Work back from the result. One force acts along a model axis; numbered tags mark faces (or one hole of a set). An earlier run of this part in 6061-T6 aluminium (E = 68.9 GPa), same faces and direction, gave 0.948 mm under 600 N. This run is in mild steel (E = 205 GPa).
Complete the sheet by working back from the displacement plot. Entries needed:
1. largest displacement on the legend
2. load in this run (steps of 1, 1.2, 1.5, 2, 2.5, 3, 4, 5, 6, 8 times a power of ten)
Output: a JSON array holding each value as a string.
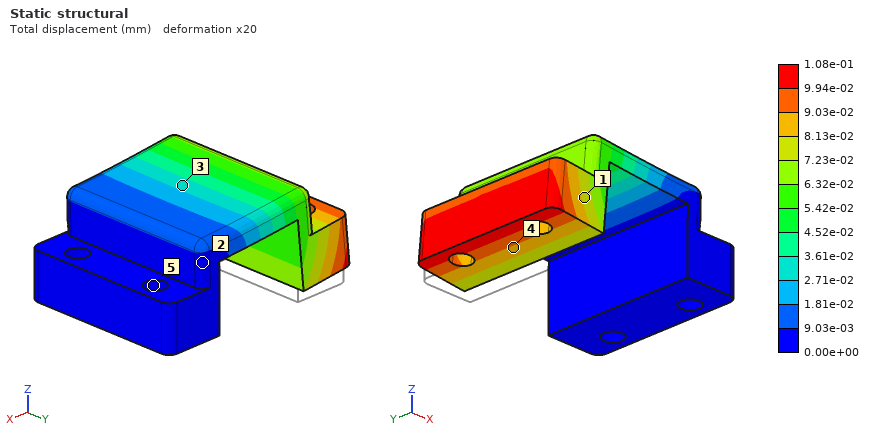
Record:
["1.08e-01 mm", "200 N"]
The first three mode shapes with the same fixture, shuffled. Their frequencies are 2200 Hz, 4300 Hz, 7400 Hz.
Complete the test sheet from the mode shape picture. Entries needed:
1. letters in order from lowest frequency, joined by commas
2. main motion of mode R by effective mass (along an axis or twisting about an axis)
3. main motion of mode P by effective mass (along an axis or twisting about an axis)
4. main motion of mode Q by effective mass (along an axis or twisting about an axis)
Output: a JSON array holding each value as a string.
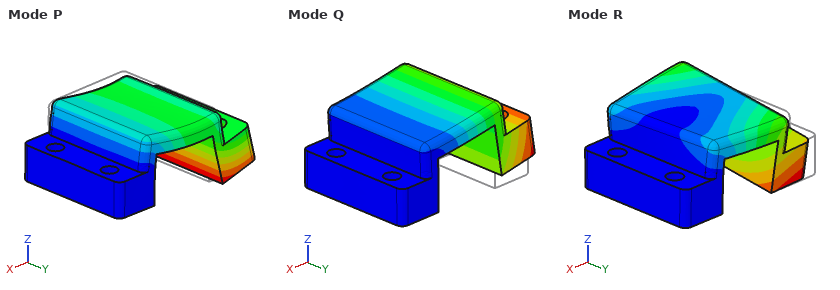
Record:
["Q, R, P", "along Y", "along X", "along Z"]
